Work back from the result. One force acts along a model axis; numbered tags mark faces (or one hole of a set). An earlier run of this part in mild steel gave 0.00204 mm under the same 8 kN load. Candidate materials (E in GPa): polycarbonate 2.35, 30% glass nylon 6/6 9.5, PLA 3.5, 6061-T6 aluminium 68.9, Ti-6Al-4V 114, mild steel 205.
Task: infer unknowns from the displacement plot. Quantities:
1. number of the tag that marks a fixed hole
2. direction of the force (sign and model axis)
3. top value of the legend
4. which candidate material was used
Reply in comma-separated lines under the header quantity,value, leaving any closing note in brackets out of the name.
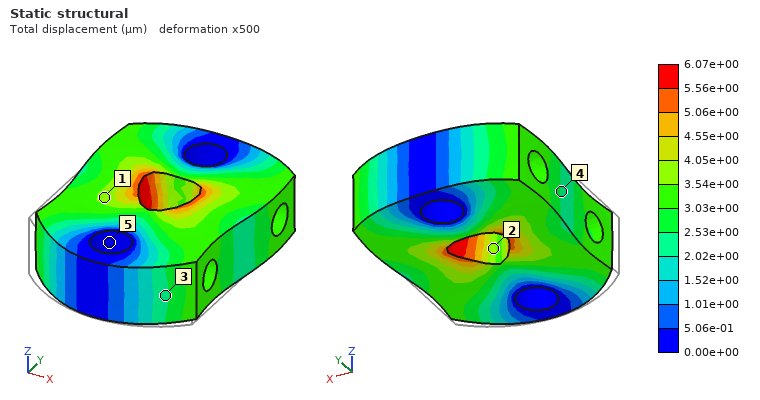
quantity,value
number of the tag that marks a fixed hole,5
direction of the force,+Y
top value of the legend,6.07e+00 µm
which candidate material was used,6061-T6 aluminium
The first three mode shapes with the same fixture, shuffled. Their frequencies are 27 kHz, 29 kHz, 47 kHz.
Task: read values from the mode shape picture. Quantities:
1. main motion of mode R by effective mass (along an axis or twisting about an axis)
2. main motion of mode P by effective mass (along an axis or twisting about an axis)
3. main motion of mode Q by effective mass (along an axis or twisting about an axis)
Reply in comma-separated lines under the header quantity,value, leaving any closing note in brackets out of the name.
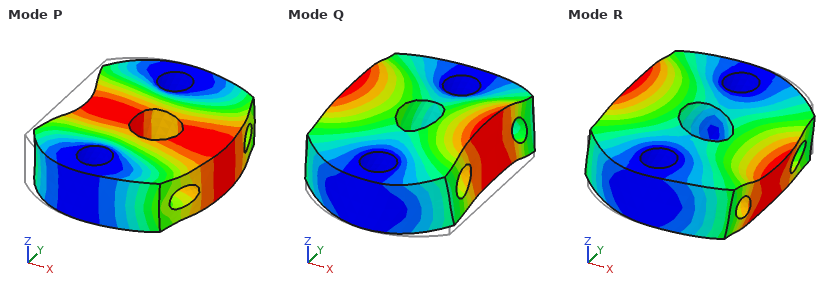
quantity,value
main motion of mode R by effective mass,twisting about Y
main motion of mode P by effective mass,along X
main motion of mode Q by effective mass,along Z
